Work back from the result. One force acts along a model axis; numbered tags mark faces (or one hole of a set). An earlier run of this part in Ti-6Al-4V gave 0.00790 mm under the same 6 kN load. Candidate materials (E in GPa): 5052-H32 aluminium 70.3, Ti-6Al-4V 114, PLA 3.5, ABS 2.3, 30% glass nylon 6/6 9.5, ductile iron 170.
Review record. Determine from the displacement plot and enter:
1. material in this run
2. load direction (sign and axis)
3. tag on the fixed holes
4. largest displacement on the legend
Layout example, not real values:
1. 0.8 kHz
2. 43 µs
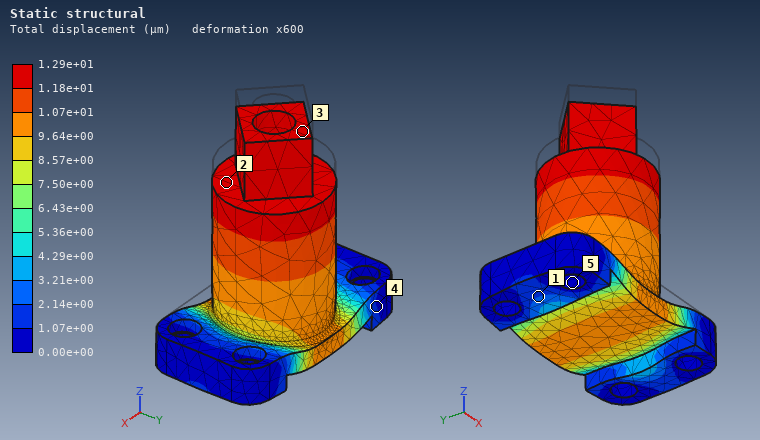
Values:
1. 5052-H32 aluminium
2. -Z
3. 5
4. 1.29e+01 µm
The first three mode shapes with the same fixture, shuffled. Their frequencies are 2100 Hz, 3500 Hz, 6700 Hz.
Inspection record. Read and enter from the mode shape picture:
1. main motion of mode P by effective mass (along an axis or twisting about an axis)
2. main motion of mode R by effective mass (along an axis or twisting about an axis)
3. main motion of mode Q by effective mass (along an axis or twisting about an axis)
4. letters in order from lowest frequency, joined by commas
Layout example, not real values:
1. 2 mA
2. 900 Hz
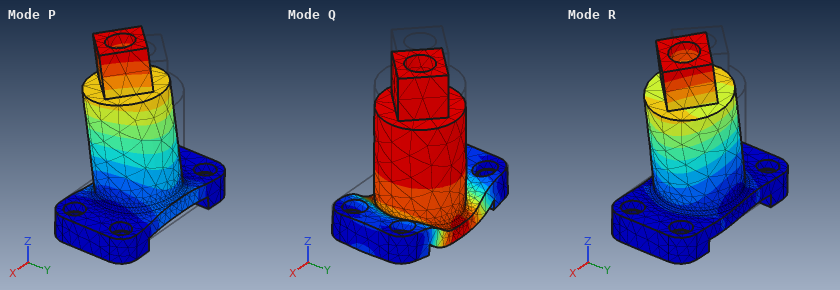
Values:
1. along Y
2. along X
3. along Z
4. P, R, Q
